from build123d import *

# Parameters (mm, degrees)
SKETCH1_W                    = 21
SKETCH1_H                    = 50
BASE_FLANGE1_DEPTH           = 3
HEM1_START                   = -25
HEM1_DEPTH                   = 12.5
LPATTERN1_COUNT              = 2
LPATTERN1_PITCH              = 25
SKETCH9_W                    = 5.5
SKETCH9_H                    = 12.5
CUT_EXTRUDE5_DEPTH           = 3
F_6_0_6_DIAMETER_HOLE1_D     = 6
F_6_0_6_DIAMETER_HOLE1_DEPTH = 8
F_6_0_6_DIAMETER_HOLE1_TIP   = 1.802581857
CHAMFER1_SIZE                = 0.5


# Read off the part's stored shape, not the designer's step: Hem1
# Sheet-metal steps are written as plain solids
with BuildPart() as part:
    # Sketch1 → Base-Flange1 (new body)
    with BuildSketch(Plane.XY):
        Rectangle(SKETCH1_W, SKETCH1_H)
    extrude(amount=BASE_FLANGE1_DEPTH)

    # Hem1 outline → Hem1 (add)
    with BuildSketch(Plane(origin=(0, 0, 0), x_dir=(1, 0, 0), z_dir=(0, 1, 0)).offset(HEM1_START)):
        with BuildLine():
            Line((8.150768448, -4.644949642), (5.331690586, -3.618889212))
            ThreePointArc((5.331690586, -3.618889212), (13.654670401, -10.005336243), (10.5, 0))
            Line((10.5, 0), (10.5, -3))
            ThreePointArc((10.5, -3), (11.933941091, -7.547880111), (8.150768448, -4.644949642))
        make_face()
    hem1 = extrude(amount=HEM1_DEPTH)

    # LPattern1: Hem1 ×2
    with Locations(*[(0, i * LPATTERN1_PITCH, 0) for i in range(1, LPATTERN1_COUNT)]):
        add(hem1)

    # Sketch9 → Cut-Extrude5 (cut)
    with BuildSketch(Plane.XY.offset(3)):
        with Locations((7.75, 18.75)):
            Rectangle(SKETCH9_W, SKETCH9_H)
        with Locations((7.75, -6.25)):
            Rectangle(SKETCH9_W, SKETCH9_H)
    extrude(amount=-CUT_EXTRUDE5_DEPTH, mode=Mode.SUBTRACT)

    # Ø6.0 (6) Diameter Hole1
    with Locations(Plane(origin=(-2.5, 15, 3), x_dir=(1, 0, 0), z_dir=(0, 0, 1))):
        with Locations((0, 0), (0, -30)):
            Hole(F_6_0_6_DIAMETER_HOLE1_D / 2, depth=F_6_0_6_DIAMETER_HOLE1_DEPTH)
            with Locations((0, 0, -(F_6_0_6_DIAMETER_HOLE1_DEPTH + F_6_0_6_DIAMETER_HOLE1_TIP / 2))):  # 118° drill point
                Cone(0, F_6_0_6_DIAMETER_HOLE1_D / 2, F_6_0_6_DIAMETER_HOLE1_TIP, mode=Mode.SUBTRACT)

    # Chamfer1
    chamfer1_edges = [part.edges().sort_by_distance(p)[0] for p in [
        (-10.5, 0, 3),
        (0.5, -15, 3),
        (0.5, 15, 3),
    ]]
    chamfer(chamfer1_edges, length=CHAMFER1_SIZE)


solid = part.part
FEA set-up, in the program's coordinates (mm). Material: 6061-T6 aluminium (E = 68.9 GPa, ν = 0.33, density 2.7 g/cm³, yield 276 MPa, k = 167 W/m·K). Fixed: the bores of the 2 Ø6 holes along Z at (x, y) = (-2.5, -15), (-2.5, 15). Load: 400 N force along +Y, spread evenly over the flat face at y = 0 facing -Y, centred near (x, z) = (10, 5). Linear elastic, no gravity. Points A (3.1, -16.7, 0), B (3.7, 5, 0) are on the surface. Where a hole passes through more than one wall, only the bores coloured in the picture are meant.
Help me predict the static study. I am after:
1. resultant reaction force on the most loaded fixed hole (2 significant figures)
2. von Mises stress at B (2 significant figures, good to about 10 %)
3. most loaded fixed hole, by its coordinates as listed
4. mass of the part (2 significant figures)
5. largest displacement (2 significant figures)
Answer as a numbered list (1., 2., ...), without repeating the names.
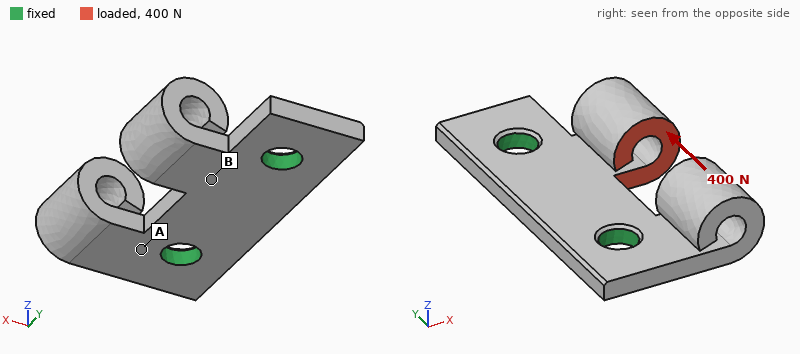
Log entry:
1. 320 N
2. 36 MPa
3. (-2.5, 15)
4. 11 g
5. 93 µm
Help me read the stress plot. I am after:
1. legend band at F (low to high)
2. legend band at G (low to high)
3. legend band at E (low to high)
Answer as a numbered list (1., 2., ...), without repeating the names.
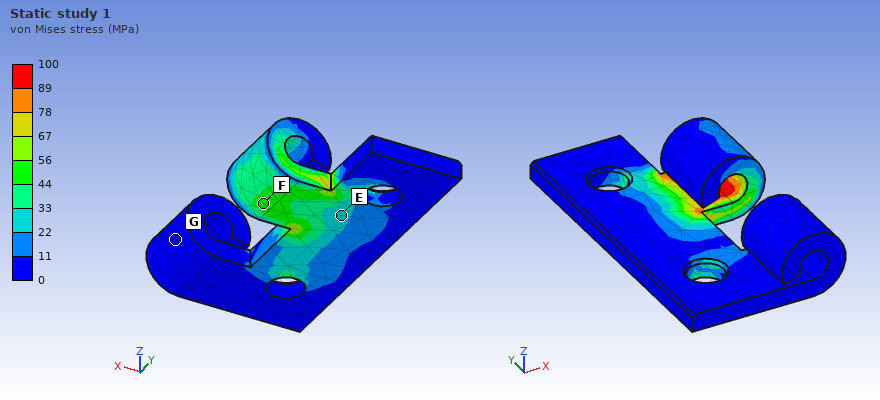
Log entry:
1. 44 to 56 MPa
2. 0 to 11 MPa
3. 22 to 33 MPa
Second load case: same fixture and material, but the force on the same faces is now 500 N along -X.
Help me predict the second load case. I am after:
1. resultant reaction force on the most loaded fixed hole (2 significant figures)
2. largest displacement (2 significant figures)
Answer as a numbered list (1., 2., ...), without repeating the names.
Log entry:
1. 260 N
2. 0.19 mm
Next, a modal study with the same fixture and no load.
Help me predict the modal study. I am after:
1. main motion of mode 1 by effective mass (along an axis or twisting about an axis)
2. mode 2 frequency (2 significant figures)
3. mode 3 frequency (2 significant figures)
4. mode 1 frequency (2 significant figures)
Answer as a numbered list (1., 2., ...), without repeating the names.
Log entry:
1. along Z
2. 4800 Hz
3. 6800 Hz
4. 4600 Hz
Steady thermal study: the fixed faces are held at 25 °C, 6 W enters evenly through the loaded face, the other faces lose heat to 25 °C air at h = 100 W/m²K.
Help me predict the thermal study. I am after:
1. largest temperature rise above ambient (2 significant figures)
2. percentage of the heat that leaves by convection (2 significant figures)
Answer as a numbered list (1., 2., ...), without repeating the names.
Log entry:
1. 17 K
2. 18 %
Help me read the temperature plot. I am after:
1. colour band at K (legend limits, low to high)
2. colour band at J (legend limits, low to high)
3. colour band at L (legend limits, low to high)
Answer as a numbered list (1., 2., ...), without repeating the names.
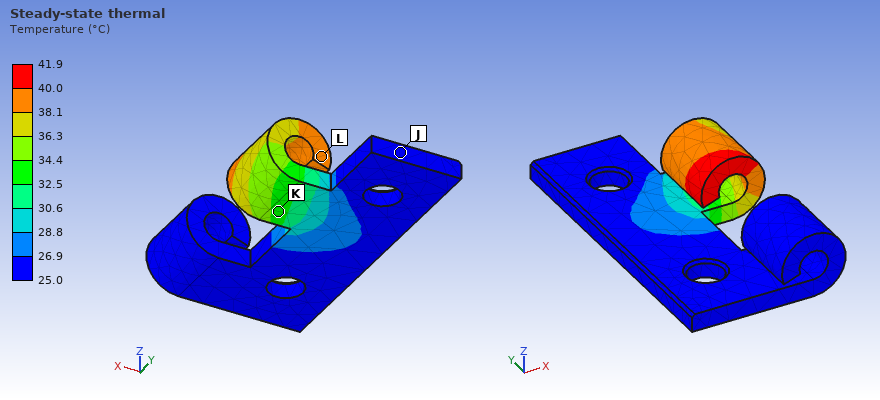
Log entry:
1. 32.5 to 34.4 °C
2. 25.0 to 26.9 °C
3. 38.1 to 40.0 °C
